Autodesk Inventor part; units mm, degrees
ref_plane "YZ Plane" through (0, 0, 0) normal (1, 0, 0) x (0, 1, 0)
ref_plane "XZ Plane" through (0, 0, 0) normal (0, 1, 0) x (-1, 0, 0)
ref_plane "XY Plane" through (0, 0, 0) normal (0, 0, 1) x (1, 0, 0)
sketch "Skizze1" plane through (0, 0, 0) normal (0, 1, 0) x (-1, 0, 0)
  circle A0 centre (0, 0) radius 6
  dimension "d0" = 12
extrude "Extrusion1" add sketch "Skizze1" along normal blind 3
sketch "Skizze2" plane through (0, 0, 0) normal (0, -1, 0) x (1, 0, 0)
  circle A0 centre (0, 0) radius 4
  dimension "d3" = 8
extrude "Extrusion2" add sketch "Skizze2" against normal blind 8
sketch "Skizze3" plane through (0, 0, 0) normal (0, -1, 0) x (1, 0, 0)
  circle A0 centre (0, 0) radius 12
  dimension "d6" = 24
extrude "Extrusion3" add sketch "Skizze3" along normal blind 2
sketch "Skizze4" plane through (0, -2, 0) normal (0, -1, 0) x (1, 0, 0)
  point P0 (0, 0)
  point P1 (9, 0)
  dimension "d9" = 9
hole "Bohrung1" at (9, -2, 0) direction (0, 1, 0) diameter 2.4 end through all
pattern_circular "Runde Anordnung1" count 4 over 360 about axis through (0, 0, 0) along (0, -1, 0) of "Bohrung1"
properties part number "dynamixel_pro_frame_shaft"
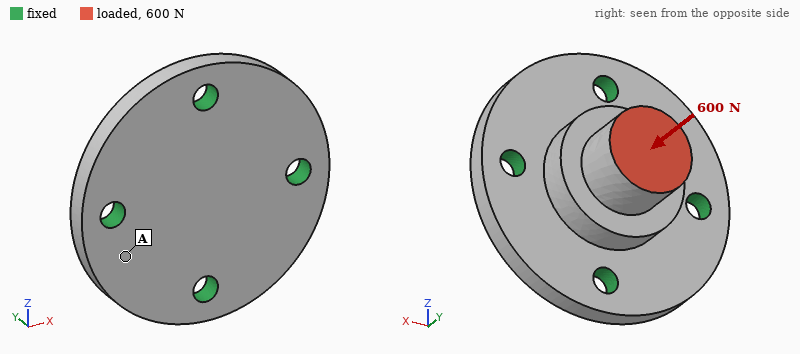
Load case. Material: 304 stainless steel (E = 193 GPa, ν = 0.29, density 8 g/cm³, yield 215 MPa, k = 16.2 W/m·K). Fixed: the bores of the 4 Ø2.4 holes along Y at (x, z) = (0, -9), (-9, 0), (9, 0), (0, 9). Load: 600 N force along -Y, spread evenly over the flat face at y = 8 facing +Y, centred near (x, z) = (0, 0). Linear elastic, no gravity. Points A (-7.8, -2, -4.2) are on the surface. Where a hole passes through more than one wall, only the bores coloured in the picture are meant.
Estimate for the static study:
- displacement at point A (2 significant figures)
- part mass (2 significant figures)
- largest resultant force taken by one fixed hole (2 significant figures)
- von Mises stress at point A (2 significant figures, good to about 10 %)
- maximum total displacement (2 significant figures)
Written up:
0.48 µm
12 g
160 N
10.0 MPa
1.7 µm
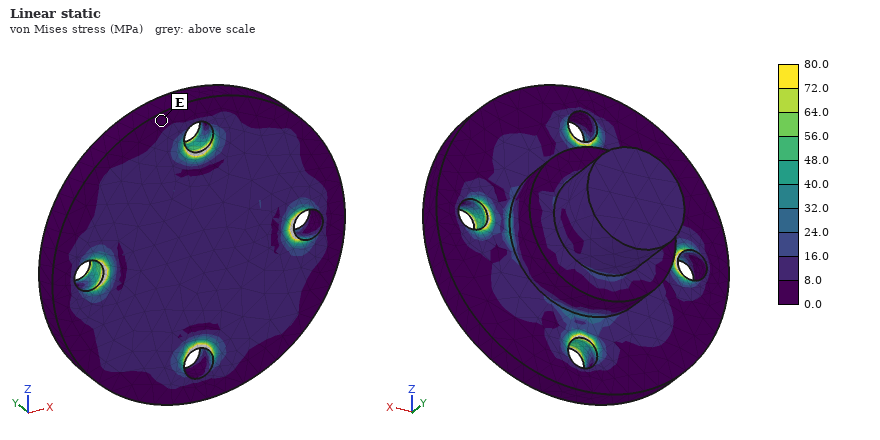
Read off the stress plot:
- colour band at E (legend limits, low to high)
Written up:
0.0 to 8.0 MPa
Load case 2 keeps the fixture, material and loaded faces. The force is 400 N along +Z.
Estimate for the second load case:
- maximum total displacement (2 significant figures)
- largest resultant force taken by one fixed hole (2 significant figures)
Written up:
4.5 µm
270 N
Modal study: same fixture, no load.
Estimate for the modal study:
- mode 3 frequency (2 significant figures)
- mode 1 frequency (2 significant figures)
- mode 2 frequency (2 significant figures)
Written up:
40 kHz
39 kHz
39 kHz
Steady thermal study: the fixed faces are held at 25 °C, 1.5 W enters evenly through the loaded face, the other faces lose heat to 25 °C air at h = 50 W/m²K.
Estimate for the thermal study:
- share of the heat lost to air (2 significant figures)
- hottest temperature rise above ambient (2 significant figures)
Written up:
15 %
18 K
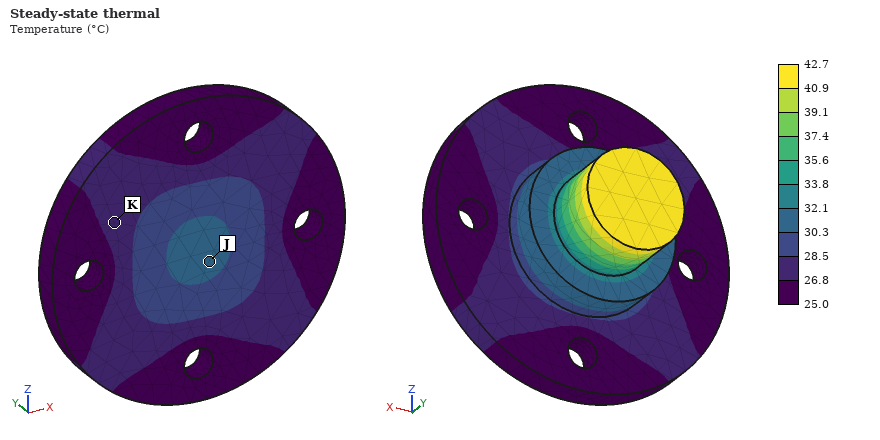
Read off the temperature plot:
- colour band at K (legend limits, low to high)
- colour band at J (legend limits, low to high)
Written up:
26.8 to 28.5 °C
30.3 to 32.1 °C
